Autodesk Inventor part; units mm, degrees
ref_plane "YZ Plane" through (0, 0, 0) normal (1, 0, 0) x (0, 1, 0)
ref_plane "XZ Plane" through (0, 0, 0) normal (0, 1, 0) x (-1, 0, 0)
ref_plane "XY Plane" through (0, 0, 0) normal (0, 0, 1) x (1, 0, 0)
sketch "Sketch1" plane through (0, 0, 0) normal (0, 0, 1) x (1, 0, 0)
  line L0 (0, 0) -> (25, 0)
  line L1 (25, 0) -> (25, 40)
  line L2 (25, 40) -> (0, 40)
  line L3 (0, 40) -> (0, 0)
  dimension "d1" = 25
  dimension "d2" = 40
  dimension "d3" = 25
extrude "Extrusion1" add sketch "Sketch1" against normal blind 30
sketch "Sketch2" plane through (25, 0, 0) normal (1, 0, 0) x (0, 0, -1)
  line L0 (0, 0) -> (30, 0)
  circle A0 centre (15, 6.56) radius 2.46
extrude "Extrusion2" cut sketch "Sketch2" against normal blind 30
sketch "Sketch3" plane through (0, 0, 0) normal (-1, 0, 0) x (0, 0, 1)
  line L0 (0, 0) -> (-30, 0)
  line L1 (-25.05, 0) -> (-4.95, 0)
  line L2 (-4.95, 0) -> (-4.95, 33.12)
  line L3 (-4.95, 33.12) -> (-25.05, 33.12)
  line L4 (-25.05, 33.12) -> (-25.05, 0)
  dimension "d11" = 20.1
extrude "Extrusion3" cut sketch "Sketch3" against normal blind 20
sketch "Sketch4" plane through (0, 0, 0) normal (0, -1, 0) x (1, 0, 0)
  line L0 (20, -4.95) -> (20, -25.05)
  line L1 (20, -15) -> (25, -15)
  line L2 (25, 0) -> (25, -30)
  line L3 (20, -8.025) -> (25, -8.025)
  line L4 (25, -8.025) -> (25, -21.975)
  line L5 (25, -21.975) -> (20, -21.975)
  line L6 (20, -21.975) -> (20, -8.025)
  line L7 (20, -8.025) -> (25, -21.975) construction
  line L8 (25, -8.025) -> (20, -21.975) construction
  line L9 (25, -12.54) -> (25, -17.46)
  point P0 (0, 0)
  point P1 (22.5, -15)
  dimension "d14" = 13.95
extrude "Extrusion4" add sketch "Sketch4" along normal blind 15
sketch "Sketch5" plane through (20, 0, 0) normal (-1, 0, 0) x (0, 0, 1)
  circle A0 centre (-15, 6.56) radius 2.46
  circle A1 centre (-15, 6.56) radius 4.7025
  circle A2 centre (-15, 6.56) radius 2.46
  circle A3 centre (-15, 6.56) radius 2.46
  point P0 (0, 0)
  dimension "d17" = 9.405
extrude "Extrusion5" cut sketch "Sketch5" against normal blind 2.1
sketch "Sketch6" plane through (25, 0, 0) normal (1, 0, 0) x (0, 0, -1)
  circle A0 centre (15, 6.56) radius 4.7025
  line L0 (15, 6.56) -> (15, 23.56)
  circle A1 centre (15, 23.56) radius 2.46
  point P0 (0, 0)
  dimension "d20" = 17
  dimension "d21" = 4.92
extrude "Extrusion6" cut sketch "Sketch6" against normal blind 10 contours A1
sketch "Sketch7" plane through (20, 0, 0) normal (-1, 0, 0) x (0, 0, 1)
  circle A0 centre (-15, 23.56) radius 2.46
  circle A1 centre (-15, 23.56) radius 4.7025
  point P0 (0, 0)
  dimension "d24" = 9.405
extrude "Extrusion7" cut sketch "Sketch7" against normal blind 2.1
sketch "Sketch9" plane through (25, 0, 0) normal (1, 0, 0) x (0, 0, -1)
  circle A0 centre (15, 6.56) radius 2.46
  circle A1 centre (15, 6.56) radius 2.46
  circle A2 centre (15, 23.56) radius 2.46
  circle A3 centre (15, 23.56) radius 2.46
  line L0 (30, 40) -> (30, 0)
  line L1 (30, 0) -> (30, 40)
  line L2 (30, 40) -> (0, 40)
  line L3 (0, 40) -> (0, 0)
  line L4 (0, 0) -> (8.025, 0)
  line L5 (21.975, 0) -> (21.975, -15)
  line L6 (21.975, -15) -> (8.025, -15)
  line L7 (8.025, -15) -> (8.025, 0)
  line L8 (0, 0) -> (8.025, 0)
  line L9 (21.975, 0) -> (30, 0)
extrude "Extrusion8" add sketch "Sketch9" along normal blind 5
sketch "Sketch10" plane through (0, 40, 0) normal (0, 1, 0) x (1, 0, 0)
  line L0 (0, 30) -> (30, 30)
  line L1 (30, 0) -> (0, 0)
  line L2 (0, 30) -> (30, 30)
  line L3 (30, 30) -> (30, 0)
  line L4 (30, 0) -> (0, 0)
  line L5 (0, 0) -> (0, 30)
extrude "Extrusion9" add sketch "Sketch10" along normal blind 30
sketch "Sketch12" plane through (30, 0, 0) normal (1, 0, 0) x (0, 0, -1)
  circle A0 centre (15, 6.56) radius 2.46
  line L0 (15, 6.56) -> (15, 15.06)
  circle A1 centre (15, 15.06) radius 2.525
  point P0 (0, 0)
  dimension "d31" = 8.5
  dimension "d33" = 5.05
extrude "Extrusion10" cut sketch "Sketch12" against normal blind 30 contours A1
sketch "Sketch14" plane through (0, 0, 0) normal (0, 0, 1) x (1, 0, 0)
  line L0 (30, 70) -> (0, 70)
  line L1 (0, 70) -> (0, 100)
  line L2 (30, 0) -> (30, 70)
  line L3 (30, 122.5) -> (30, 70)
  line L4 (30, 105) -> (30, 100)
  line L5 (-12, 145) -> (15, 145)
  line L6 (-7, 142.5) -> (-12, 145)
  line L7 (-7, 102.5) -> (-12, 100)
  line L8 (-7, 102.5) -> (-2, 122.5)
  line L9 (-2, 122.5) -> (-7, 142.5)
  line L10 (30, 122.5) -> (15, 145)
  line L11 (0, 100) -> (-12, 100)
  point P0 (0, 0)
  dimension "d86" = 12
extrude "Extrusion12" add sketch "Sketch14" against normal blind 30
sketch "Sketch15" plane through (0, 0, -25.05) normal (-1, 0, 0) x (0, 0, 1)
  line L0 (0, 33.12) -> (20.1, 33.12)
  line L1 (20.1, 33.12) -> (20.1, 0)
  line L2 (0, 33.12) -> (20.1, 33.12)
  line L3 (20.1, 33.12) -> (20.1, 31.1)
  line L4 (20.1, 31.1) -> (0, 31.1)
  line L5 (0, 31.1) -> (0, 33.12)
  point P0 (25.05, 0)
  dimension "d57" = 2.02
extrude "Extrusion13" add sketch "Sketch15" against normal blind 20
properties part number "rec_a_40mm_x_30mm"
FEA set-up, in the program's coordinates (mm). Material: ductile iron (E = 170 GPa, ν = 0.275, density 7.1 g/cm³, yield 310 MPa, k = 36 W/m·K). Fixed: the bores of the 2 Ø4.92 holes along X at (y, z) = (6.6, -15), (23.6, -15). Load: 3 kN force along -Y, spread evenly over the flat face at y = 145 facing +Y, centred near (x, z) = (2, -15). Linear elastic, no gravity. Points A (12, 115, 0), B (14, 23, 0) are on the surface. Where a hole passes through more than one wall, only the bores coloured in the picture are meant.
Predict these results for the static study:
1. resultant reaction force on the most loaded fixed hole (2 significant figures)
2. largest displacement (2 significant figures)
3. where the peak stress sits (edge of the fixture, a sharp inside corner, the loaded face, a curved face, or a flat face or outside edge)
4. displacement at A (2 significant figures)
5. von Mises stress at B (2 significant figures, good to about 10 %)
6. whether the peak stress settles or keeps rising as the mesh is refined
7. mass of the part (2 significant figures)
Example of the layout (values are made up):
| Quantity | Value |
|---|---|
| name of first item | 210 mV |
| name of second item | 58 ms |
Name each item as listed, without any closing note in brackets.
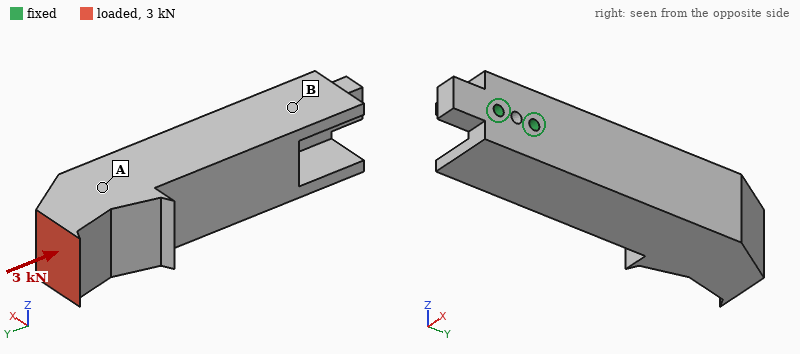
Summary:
| Quantity | Value |
|---|---|
| resultant reaction force on the most loaded fixed hole | 3.4 kN |
| largest displacement | 0.11 mm |
| where the peak stress sits | edge of the fixture |
| displacement at A | 0.071 mm |
| von Mises stress at B | 21 MPa |
| whether the peak stress settles or keeps rising as the mesh is refined | keeps rising |
| mass of the part | 860 g |
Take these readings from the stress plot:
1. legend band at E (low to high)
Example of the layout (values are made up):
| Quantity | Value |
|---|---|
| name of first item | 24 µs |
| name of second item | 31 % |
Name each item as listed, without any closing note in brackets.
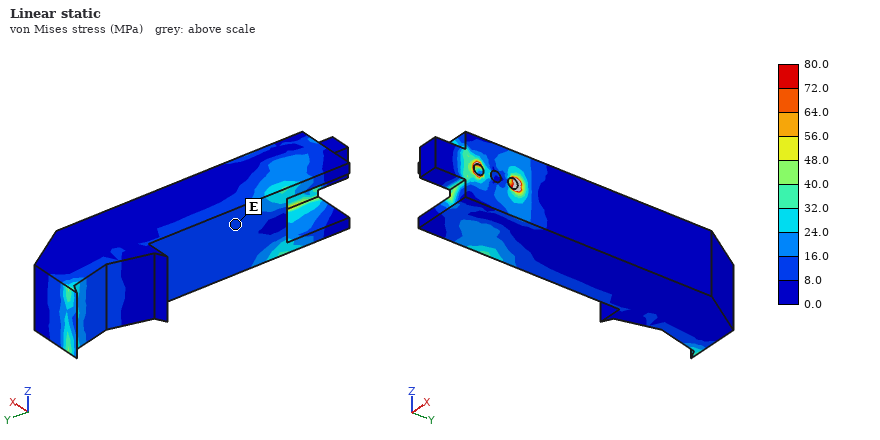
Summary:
| Quantity | Value |
|---|---|
| legend band at E | 8.0 to 16.0 MPa |
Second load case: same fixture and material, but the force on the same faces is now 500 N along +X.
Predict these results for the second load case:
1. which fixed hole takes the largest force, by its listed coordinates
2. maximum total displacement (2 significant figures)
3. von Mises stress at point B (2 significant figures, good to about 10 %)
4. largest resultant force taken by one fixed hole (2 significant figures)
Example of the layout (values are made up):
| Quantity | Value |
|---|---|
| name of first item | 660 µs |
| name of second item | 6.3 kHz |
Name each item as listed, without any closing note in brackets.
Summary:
| Quantity | Value |
|---|---|
| which fixed hole takes the largest force, by its listed coordinates | (23.6, -15) |
| maximum total displacement | 93 µm |
| von Mises stress at point B | 16 MPa |
| largest resultant force taken by one fixed hole | 3.0 kN |
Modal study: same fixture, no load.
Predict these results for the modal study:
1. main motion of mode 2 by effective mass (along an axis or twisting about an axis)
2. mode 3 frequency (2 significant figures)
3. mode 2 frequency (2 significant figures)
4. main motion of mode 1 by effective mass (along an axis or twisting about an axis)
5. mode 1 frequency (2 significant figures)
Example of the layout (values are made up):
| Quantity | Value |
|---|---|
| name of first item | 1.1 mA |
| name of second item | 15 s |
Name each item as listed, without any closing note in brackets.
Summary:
| Quantity | Value |
|---|---|
| main motion of mode 2 by effective mass | along Z |
| mode 3 frequency | 2800 Hz |
| mode 2 frequency | 890 Hz |
| main motion of mode 1 by effective mass | along X |
| mode 1 frequency | 760 Hz |
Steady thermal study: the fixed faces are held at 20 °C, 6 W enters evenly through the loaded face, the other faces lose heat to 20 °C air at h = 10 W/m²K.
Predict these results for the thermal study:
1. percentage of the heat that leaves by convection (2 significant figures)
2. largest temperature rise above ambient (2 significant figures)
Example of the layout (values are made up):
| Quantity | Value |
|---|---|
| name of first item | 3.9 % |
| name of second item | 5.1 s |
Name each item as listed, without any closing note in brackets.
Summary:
| Quantity | Value |
|---|---|
| percentage of the heat that leaves by convection | 33 % |
| largest temperature rise above ambient | 26 K |
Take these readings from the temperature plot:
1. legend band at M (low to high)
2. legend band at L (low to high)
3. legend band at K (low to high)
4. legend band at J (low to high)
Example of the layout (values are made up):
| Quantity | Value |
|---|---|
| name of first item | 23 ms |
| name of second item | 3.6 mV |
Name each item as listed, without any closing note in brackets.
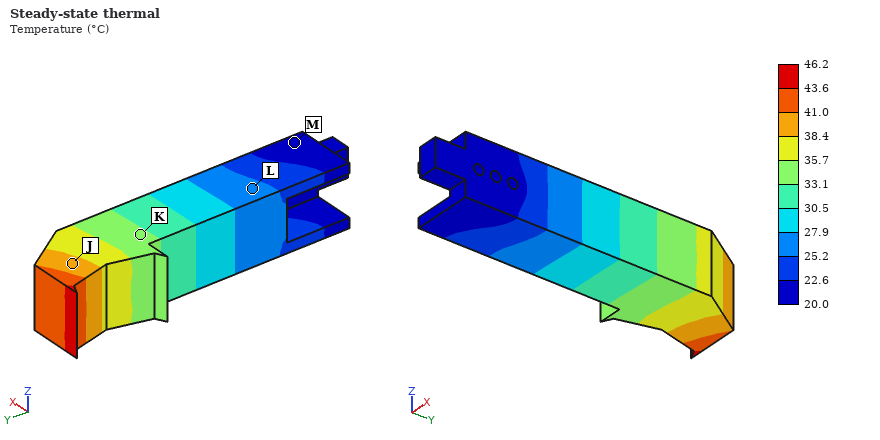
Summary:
| Quantity | Value |
|---|---|
| legend band at M | 20.0 to 22.6 °C |
| legend band at L | 25.2 to 27.9 °C |
| legend band at K | 33.1 to 35.7 °C |
| legend band at J | 38.4 to 41.0 °C |
